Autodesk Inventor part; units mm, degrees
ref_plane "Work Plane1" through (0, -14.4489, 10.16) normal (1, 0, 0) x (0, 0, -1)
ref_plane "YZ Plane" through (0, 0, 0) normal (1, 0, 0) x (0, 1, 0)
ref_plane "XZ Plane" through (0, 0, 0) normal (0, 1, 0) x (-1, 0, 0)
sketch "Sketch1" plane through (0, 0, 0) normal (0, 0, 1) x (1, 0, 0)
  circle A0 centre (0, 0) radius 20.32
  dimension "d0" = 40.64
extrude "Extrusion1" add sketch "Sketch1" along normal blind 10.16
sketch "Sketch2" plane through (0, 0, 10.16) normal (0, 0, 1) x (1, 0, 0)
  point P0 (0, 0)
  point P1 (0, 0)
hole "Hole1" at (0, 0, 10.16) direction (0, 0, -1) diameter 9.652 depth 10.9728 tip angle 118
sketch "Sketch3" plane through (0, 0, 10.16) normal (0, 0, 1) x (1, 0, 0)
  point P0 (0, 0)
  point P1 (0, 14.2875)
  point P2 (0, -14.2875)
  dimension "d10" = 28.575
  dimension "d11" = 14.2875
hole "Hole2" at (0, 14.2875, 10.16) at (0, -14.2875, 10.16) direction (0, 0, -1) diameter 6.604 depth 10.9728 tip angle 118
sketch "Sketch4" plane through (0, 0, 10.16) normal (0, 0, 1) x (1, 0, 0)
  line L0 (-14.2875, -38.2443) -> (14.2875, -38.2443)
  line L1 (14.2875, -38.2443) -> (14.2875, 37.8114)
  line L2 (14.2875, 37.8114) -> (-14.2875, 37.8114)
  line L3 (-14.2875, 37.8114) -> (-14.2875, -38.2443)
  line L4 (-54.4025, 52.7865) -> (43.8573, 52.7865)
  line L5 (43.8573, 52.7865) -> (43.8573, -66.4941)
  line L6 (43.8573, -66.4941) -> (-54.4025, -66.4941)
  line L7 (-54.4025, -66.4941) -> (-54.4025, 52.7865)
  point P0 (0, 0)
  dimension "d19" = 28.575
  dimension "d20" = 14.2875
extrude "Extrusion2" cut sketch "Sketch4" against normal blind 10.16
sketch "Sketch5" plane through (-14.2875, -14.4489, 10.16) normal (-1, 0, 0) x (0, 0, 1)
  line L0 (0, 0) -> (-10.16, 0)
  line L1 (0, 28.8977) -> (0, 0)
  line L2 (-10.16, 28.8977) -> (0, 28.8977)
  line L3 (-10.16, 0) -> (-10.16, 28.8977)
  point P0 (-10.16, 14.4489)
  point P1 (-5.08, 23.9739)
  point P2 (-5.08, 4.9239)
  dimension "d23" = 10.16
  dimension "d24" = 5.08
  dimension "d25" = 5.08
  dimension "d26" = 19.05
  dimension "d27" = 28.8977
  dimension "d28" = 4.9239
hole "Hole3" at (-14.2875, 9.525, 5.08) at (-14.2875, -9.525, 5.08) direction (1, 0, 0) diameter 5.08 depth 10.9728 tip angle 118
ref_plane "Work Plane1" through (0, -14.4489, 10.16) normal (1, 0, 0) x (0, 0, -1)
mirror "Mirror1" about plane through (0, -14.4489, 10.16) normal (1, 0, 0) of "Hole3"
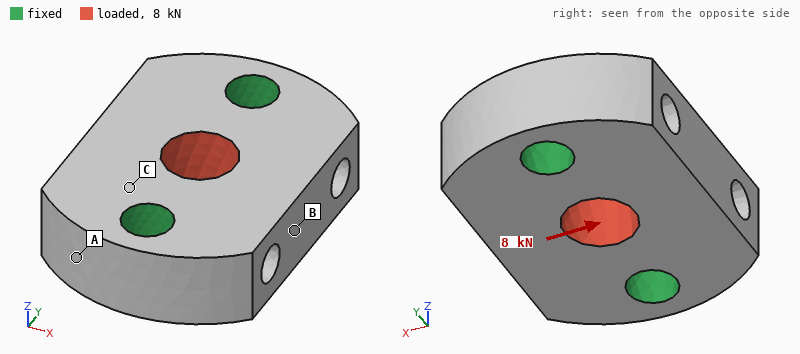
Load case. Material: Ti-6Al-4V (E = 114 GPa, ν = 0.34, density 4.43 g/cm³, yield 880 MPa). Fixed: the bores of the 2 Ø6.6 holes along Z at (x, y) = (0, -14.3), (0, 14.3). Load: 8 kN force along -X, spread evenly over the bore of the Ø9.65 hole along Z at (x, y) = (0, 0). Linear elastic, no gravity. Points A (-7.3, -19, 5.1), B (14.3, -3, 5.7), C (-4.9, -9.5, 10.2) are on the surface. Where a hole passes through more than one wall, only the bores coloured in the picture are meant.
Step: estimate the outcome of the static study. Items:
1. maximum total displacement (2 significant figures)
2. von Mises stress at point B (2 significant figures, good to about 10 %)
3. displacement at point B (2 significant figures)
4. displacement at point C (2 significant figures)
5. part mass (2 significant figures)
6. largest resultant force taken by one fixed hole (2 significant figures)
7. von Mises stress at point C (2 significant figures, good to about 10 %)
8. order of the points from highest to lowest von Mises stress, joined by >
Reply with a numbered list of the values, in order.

1. 6.5 µm
2. 24 MPa
3. 4.9 µm
4. 2.3 µm
5. 37 g
6. 4.0 kN
7. 44 MPa
8. C > B > A
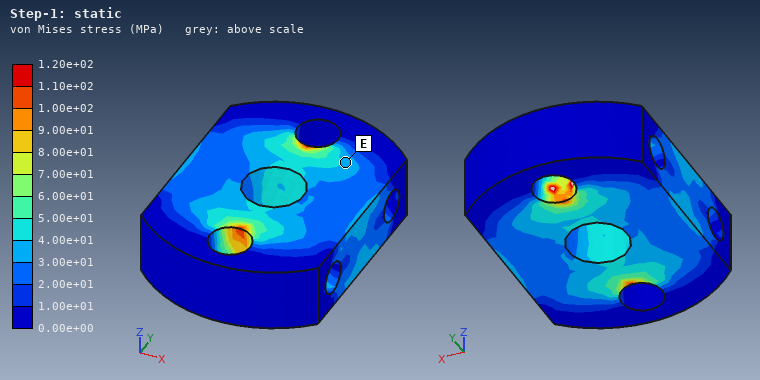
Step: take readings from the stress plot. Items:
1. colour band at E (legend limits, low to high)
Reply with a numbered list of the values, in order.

1. 3.00e+01 to 4.00e+01 MPa
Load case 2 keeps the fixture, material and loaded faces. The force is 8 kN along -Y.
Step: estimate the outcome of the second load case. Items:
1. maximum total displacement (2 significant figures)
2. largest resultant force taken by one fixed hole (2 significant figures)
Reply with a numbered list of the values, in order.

1. 3.7 µm
2. 4.0 kN
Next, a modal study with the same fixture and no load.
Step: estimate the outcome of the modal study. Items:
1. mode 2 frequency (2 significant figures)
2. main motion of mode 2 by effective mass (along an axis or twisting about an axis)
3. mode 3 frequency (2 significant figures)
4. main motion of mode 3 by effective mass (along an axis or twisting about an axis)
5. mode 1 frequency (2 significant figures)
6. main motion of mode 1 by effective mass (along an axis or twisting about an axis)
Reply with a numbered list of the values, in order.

1. 29 kHz
2. along Z
3. 47 kHz
4. along X
5. 27 kHz
6. twisting about Y
